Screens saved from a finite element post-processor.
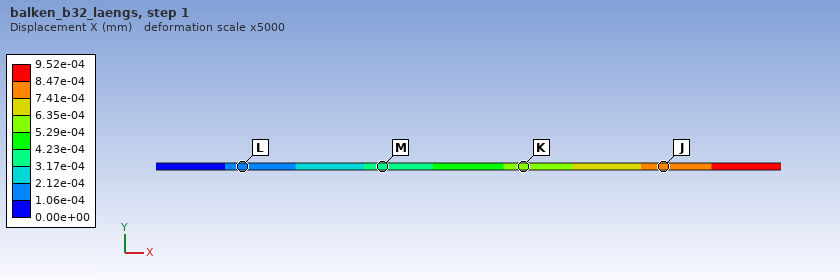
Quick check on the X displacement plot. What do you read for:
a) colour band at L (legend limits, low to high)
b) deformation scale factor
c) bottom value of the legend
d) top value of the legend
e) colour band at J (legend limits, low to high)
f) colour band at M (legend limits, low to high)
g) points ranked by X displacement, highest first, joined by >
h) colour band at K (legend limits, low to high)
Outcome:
1.06e-04 to 2.12e-04 mm
5000
0.00e+00 mm
9.52e-04 mm
7.41e-04 to 8.47e-04 mm
3.17e-04 to 4.23e-04 mm
J > K > M > L
5.29e-04 to 6.35e-04 mm
